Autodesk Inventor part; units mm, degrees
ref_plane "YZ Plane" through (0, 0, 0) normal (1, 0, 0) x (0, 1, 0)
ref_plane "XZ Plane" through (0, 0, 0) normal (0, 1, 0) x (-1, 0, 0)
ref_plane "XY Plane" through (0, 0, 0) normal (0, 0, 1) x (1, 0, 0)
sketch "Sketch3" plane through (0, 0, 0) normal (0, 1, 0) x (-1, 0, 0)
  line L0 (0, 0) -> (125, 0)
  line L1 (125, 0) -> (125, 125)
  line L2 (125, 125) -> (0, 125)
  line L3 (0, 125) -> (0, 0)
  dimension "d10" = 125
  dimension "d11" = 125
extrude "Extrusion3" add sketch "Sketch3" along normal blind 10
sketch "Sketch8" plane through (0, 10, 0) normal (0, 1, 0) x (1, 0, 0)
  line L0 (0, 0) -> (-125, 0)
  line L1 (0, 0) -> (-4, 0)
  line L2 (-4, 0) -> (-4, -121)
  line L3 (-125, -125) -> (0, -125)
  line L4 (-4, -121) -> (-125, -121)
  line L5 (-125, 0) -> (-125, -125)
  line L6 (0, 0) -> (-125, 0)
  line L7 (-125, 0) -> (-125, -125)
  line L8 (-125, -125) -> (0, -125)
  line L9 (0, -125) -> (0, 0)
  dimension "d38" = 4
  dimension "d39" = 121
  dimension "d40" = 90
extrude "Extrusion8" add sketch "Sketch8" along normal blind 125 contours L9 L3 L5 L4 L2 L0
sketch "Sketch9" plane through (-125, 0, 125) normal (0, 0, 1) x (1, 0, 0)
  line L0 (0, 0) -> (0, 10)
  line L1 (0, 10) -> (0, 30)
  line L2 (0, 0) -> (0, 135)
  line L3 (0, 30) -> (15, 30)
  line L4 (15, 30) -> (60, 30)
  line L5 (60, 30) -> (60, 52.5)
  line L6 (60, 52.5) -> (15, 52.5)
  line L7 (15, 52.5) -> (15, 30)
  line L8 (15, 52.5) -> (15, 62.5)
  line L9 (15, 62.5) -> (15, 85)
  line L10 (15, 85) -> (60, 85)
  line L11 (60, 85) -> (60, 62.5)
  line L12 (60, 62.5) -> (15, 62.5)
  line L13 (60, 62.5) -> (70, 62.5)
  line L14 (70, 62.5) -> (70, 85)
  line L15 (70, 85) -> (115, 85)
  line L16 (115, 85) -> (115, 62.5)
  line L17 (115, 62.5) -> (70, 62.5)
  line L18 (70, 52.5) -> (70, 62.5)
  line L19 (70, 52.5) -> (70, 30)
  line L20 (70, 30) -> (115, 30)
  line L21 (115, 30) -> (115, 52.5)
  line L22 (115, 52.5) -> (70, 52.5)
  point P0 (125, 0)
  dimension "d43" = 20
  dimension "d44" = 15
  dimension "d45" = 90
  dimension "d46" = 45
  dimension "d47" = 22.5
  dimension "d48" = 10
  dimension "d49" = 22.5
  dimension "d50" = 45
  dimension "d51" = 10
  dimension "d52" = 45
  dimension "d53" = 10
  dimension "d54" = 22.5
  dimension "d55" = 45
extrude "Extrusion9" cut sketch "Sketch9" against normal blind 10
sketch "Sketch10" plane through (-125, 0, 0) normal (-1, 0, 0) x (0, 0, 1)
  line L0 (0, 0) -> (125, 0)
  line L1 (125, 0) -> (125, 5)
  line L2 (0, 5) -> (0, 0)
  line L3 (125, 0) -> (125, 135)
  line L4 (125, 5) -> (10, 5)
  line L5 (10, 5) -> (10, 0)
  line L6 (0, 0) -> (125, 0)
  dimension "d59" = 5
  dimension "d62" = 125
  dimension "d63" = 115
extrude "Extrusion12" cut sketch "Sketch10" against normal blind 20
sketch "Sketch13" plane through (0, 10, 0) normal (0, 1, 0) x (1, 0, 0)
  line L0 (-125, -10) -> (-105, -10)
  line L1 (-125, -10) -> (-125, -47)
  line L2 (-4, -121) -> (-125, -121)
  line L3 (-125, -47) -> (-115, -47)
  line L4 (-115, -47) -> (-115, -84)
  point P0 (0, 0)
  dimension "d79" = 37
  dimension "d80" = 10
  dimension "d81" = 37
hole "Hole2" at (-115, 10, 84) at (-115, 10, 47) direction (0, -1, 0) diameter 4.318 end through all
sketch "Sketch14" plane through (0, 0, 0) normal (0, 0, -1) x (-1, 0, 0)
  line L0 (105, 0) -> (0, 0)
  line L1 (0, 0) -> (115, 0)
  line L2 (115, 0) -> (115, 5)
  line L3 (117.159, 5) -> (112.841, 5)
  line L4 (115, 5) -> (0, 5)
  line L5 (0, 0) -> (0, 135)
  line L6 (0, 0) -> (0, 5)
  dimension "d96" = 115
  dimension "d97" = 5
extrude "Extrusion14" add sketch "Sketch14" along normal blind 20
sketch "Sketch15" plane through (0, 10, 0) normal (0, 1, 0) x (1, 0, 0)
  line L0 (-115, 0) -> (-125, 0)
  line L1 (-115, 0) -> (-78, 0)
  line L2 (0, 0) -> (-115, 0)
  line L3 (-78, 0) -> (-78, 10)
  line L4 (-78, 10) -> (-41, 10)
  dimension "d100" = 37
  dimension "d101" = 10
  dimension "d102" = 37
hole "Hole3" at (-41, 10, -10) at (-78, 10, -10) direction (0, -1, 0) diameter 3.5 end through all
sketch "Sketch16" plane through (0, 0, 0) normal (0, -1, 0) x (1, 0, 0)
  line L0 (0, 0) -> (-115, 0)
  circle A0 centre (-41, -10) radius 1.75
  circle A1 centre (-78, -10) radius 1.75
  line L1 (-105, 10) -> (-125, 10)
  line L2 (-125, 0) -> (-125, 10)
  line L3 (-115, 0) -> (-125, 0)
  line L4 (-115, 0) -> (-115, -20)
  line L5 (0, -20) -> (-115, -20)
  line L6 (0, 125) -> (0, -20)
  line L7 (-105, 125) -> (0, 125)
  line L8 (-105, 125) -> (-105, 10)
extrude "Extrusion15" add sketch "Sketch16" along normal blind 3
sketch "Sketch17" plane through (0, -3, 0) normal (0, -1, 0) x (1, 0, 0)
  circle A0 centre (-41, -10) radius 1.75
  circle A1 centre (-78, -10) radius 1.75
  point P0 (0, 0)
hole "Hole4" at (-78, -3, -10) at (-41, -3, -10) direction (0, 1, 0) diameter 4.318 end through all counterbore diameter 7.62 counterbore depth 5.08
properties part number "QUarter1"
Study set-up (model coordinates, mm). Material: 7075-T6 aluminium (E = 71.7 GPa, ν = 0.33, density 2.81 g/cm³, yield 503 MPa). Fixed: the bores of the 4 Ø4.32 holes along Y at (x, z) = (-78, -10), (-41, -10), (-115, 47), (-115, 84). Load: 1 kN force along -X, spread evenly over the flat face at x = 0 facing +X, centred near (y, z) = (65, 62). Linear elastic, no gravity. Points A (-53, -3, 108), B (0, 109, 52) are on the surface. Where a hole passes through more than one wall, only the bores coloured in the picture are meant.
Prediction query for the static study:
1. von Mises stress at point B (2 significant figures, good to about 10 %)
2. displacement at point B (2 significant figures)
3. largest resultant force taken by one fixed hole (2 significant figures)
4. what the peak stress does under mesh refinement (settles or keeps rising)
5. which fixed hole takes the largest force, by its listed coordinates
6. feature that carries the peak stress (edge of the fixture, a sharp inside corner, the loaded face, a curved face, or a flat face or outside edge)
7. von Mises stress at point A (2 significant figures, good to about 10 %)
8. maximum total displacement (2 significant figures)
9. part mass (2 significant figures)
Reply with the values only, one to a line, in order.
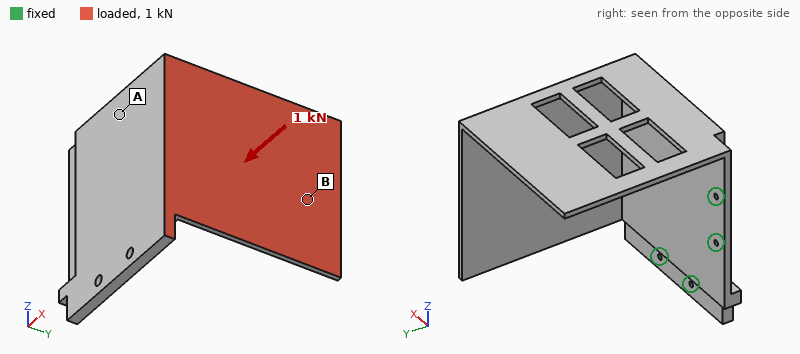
30 MPa
1.4 mm
1.3 kN
keeps rising
(-41, -10)
edge of the fixture
13 MPa
2.5 mm
870 g
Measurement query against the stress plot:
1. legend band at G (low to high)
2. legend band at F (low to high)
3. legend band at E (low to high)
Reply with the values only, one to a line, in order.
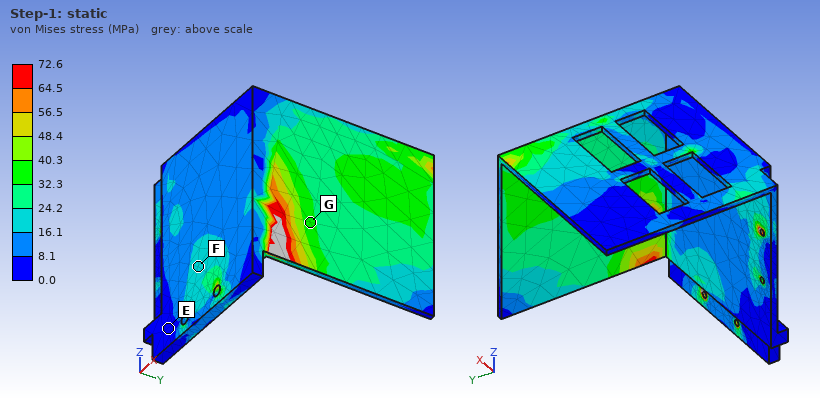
32.3 to 40.3 MPa
16.1 to 24.2 MPa
0.0 to 8.1 MPa
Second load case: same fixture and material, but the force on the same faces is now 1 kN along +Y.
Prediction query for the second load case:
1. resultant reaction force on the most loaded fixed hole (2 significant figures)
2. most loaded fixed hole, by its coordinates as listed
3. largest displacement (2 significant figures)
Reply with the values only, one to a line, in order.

2.4 kN
(-41, -10)
0.96 mm
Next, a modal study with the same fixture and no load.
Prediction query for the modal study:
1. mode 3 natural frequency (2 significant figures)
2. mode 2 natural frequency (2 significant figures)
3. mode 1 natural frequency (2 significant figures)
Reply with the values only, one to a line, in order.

450 Hz
280 Hz
250 Hz
